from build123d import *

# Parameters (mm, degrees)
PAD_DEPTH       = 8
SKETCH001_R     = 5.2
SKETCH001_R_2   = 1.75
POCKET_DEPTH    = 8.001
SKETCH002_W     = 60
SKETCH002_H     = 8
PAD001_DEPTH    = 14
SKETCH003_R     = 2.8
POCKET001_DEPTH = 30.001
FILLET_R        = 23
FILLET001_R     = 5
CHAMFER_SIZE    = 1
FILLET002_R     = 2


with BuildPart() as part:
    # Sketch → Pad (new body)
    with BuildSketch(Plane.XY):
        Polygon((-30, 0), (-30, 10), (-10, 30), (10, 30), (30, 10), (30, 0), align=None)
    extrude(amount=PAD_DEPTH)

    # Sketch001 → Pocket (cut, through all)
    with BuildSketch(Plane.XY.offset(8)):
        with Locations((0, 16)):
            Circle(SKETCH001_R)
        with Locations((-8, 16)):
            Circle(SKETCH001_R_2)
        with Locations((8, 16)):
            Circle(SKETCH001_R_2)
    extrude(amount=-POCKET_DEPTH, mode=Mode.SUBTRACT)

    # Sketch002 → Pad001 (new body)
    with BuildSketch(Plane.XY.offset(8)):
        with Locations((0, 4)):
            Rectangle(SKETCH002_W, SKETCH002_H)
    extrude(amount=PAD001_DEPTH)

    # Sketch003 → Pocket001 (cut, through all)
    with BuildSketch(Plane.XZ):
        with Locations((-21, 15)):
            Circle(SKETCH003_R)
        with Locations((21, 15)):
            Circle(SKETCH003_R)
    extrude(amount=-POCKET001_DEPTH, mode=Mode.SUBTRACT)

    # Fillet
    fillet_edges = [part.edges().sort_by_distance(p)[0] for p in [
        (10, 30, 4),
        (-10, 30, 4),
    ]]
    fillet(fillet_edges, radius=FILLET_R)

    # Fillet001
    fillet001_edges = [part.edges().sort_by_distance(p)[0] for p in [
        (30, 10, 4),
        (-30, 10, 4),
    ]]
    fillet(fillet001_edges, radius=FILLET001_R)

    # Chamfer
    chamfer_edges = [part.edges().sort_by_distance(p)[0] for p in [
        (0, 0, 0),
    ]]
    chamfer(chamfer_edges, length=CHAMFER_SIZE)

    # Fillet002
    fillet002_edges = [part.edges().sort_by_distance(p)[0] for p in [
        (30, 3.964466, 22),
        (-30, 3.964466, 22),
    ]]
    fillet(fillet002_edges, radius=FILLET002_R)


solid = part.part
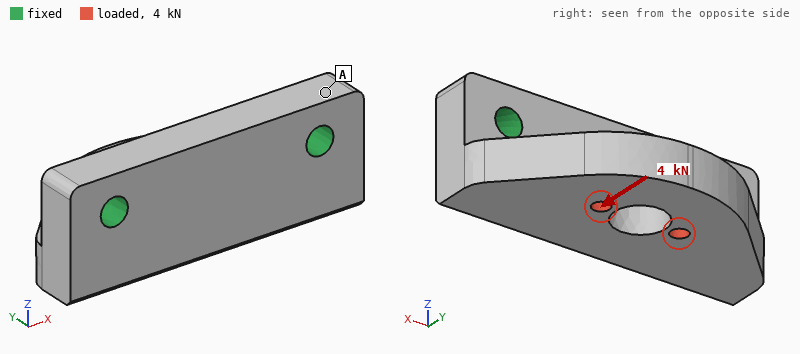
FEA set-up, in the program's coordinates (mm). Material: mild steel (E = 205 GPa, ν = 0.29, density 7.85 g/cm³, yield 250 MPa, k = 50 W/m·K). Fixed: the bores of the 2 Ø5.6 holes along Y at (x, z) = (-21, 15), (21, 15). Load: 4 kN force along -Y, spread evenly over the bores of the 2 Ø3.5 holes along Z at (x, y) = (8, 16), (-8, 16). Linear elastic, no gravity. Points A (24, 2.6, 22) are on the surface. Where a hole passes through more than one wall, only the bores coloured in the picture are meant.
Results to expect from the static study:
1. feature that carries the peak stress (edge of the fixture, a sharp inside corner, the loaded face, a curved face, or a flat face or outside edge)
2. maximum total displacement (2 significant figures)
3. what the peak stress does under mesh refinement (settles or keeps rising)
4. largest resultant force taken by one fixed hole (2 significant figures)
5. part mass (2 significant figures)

edge of the fixture
22 µm
keeps rising
2.0 kN
130 g
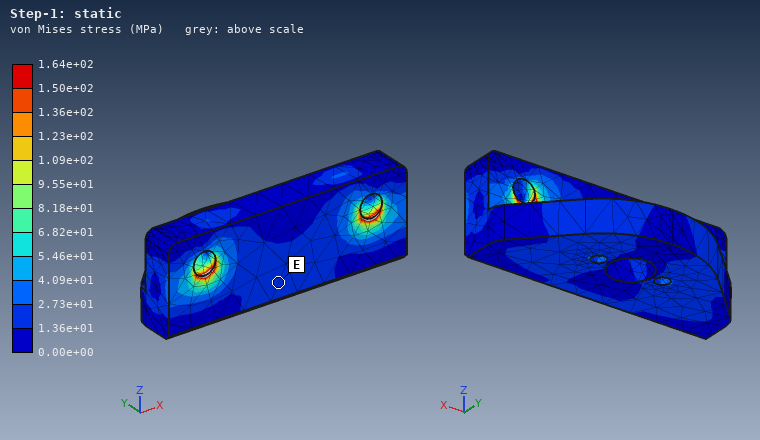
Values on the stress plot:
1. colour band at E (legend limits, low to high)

1.36e+01 to 2.73e+01 MPa
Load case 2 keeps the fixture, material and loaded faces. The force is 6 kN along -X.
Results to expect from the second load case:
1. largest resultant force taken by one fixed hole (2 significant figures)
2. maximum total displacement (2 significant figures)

3.6 kN
9.7 µm
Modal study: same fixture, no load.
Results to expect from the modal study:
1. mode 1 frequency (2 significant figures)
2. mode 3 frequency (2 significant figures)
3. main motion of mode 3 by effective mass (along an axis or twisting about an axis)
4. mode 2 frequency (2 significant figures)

7200 Hz
17 kHz
along Y
15 kHz
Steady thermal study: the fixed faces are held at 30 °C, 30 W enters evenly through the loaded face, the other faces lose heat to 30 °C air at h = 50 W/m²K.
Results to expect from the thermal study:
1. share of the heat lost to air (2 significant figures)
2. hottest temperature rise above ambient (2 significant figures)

16 %
43 K
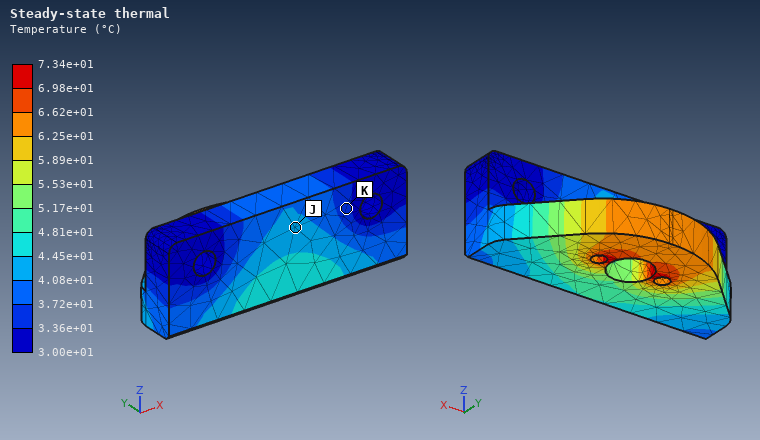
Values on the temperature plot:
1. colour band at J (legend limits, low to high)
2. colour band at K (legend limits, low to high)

4.08e+01 to 4.45e+01 °C
3.36e+01 to 3.72e+01 °C
